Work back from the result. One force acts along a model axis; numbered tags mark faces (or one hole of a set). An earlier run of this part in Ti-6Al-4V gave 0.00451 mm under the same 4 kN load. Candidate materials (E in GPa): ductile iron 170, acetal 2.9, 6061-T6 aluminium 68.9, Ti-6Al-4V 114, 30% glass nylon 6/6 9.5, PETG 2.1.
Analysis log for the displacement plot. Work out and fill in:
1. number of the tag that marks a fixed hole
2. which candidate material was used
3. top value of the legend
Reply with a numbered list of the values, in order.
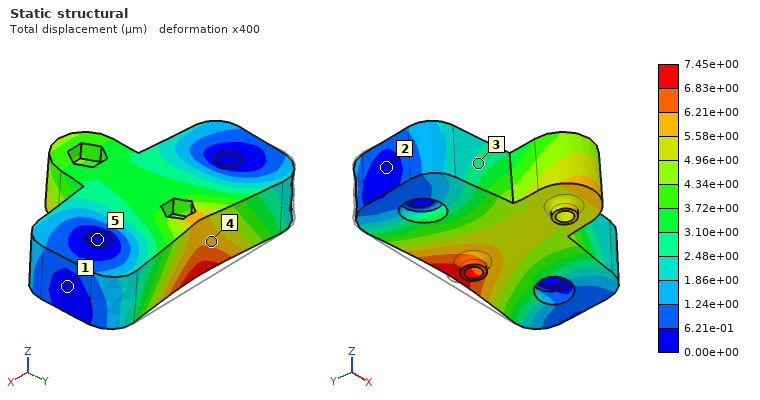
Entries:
1. 5
2. 6061-T6 aluminium
3. 7.45e+00 µm
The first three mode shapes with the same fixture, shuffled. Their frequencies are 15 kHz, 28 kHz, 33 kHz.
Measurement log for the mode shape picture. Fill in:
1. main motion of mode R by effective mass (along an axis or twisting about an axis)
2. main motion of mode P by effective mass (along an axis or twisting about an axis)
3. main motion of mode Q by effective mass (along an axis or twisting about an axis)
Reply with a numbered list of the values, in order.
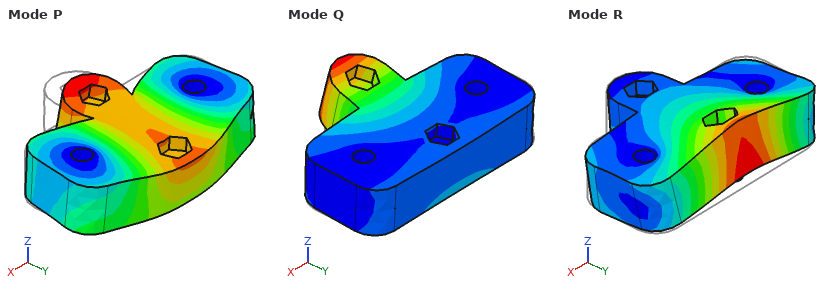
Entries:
1. along Z
2. along Y
3. along Z
